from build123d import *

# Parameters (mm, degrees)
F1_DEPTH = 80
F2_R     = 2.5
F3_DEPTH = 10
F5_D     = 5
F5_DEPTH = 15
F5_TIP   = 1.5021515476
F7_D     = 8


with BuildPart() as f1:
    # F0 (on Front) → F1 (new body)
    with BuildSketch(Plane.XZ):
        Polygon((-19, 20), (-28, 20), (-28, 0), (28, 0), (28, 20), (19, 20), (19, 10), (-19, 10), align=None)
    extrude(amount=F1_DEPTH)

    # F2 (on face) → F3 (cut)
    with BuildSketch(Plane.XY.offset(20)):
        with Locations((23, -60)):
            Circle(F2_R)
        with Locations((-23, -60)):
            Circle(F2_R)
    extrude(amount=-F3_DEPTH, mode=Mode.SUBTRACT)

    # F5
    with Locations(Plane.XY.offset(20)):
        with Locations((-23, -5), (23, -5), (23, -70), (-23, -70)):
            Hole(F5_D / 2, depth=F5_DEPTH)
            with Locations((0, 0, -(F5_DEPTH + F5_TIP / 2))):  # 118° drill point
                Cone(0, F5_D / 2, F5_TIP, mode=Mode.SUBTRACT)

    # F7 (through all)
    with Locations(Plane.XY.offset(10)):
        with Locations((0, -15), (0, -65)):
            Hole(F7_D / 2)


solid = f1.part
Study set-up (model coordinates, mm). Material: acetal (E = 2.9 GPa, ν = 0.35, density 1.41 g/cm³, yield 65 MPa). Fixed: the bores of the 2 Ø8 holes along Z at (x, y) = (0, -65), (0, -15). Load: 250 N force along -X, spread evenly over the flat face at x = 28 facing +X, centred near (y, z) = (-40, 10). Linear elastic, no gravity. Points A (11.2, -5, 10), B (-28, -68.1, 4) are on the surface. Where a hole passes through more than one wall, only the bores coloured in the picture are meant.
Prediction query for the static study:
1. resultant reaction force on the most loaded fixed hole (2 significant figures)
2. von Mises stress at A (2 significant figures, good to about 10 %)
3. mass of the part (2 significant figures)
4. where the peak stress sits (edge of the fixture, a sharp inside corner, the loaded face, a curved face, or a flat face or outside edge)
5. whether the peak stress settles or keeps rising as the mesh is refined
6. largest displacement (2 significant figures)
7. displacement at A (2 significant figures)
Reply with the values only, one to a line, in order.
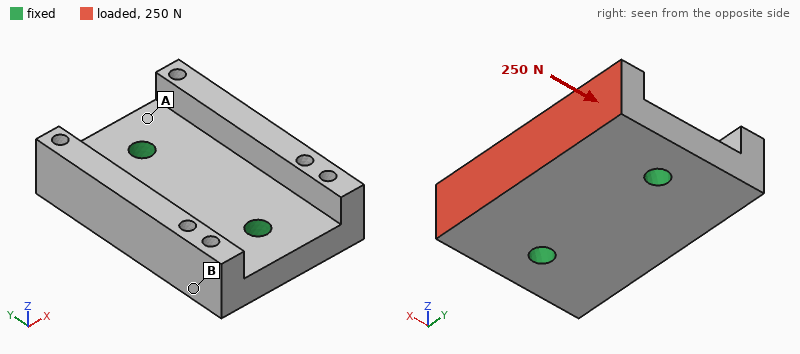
130 N
1.1 MPa
80 g
edge of the fixture
keeps rising
40 µm
6.8 µm
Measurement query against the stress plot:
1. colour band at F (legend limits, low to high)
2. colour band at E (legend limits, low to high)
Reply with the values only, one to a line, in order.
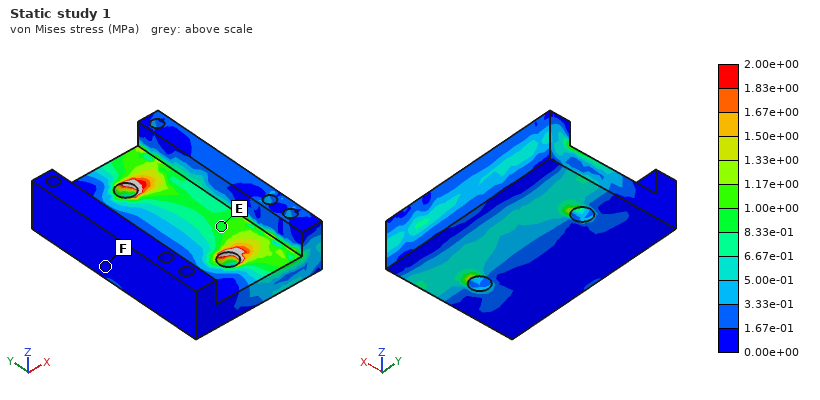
0.00e+00 to 1.67e-01 MPa
8.33e-01 to 1.00e+00 MPa
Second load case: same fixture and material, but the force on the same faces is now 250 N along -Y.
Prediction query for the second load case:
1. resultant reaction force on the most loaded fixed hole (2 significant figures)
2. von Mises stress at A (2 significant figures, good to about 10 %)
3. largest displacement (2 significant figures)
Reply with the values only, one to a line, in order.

180 N
0.42 MPa
22 µm
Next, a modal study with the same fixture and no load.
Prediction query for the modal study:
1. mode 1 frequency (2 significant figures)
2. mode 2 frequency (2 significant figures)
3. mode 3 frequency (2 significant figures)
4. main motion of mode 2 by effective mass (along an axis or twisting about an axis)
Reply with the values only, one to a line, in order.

1700 Hz
2100 Hz
2500 Hz
along Z
